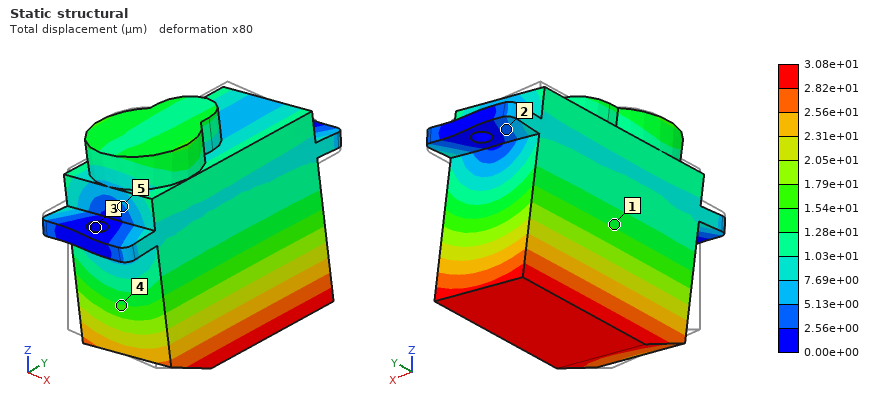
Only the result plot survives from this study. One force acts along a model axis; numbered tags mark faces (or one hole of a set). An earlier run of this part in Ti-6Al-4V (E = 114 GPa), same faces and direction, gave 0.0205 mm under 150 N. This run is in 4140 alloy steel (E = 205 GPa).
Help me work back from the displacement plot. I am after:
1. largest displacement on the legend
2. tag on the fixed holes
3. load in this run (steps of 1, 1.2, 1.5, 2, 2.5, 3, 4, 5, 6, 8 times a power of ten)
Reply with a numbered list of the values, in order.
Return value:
1. 3.08e+01 µm
2. 3
3. 400 N
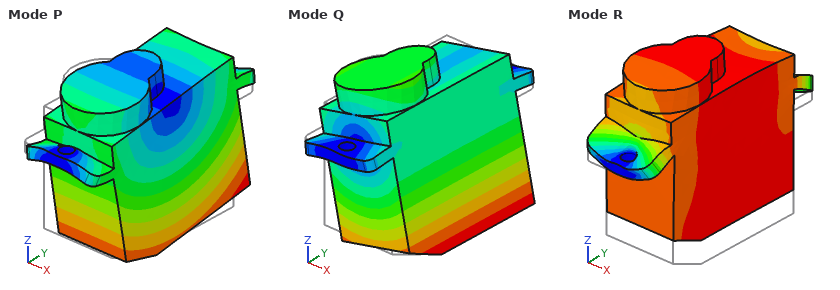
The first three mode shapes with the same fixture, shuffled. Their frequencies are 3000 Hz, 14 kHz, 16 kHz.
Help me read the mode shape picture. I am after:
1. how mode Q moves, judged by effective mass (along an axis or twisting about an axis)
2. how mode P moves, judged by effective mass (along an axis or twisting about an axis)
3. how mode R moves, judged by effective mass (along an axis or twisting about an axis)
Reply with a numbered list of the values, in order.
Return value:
1. along X
2. along Y
3. along Z
